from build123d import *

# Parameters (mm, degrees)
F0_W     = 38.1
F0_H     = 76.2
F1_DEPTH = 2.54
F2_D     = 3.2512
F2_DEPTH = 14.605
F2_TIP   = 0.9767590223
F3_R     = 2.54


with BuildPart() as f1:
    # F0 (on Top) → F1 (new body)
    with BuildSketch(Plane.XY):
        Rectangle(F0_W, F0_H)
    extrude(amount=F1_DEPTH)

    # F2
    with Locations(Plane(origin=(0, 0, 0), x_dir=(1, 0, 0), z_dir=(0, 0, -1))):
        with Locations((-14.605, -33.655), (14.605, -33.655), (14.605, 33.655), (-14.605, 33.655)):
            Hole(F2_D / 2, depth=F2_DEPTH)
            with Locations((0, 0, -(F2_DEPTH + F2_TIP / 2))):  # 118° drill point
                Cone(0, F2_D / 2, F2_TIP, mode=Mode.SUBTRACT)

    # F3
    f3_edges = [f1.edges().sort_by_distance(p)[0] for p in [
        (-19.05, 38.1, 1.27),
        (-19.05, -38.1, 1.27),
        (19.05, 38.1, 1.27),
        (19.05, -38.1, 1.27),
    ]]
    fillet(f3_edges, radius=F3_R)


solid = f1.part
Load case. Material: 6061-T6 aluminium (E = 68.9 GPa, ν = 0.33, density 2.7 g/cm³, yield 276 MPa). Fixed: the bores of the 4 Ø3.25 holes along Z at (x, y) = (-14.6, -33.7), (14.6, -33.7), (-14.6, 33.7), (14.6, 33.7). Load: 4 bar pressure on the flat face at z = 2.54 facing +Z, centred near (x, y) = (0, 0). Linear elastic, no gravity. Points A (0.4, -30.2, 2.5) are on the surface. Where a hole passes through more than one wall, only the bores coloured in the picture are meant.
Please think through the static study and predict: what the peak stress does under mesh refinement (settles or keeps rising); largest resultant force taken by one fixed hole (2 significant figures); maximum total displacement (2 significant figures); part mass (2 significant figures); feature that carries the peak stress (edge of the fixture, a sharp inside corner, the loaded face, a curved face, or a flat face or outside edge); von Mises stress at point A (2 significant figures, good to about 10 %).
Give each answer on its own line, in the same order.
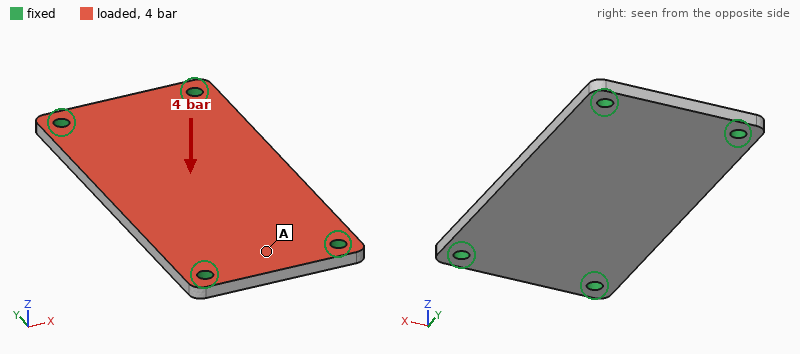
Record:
keeps rising
290 N
0.26 mm
20 g
edge of the fixture
42 MPa
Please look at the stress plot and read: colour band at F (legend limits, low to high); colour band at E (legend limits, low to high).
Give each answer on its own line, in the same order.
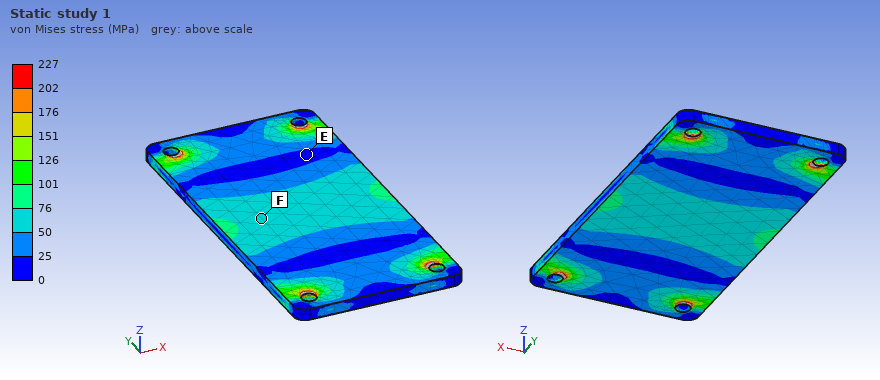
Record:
50 to 76 MPa
0 to 25 MPa
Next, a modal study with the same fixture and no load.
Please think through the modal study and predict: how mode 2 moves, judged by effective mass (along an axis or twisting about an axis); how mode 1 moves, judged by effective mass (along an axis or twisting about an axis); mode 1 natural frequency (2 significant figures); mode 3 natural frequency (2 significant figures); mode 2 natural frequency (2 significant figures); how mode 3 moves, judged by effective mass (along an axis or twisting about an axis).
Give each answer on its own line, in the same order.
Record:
twisting about Y
along Z
2700 Hz
7500 Hz
4500 Hz
twisting about X
